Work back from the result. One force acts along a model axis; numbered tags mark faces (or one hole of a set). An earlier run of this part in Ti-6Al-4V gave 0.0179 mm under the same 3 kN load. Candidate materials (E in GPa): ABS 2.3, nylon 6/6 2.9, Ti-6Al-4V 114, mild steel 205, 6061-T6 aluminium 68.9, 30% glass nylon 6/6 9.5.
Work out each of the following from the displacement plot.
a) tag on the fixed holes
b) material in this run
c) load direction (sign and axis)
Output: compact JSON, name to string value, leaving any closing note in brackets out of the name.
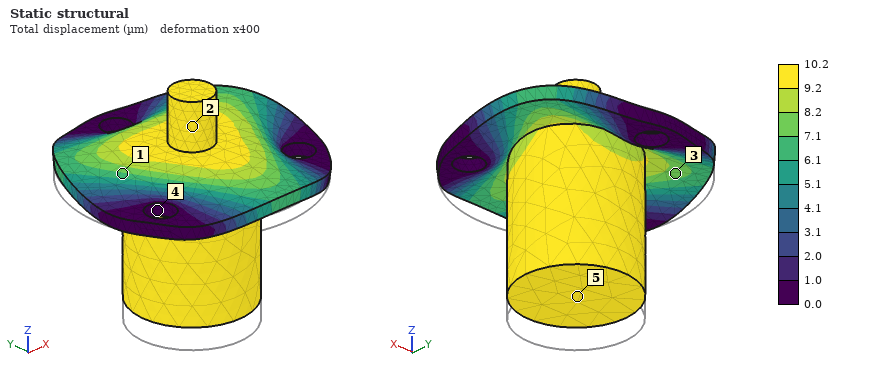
{"tag on the fixed holes": "4", "material in this run": "mild steel", "load direction": "+Z"}
